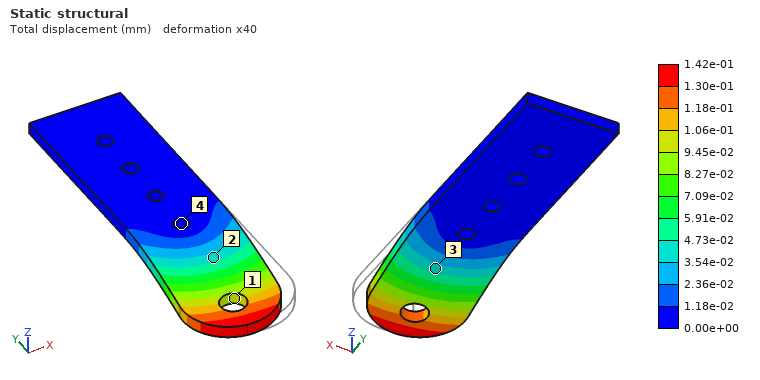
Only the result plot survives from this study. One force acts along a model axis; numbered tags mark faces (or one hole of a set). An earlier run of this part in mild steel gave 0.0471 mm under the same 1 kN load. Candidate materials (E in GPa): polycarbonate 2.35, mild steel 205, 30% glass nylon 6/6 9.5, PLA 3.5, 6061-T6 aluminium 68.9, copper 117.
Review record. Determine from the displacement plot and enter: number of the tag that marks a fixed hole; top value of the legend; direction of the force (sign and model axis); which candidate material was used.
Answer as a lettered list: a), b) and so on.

a) 4
b) 1.42e-01 mm
c) -X
d) 6061-T6 aluminium
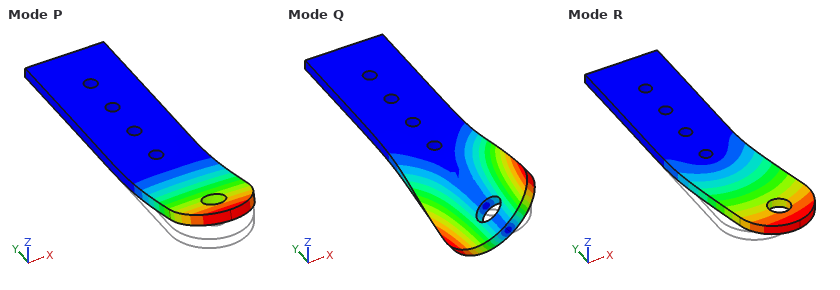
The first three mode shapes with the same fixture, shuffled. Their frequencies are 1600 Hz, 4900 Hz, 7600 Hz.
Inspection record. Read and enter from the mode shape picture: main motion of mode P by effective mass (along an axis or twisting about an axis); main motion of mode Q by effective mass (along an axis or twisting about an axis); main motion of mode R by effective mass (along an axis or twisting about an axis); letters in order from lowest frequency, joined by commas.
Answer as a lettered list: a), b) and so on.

a) along Z
b) twisting about Y
c) along X
d) P, Q, R
